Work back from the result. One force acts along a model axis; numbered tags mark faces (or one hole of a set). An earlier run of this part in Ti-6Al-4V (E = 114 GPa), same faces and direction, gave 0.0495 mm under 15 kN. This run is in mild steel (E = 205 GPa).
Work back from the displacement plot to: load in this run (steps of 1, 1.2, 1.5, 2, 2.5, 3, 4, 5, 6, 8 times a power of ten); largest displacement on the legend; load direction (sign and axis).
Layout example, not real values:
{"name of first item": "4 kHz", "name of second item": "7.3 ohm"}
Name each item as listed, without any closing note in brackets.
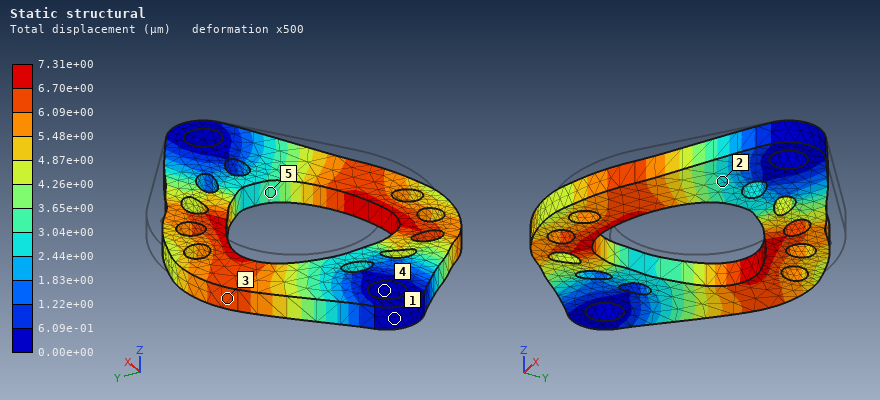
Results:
{"load in this run": "4 kN", "largest displacement on the legend": "7.31e+00 µm", "load direction": "-X"}
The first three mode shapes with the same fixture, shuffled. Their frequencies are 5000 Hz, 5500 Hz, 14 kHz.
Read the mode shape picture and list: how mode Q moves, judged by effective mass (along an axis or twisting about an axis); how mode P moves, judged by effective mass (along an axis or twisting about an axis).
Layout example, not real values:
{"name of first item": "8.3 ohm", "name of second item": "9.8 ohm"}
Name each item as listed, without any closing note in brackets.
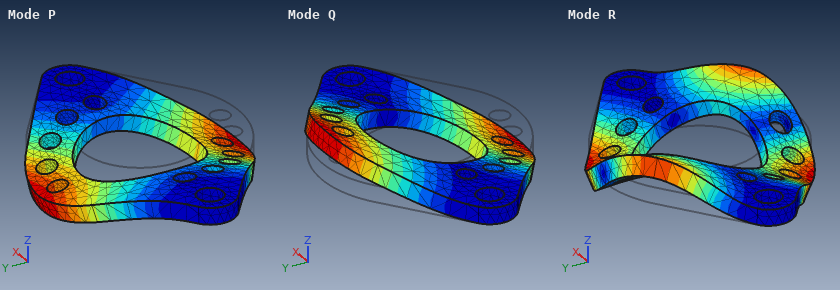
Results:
{"how mode Q moves, judged by effective mass": "twisting about X", "how mode P moves, judged by effective mass": "along Z"}
